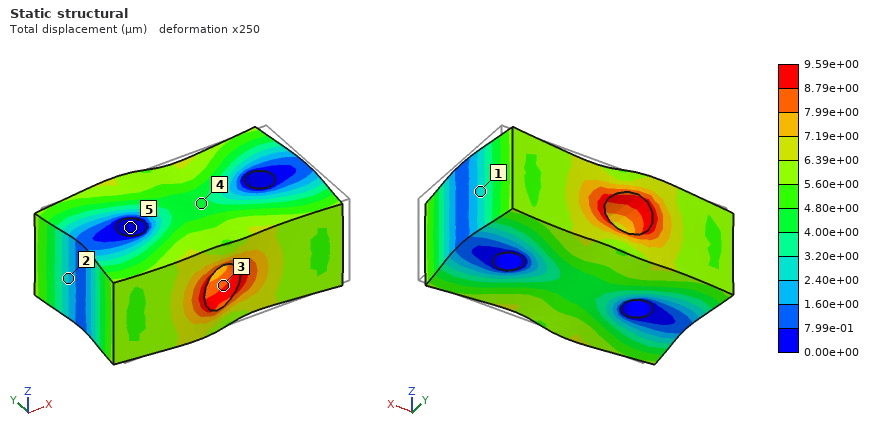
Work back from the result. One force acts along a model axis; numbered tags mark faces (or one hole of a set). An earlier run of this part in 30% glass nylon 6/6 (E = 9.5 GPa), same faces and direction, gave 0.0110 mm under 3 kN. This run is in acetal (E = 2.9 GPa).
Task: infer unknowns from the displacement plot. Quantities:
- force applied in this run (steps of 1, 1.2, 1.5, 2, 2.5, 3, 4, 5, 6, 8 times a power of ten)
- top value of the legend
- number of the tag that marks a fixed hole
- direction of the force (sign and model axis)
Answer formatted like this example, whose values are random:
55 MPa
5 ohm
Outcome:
800 N
9.59e+00 µm
5
-X
